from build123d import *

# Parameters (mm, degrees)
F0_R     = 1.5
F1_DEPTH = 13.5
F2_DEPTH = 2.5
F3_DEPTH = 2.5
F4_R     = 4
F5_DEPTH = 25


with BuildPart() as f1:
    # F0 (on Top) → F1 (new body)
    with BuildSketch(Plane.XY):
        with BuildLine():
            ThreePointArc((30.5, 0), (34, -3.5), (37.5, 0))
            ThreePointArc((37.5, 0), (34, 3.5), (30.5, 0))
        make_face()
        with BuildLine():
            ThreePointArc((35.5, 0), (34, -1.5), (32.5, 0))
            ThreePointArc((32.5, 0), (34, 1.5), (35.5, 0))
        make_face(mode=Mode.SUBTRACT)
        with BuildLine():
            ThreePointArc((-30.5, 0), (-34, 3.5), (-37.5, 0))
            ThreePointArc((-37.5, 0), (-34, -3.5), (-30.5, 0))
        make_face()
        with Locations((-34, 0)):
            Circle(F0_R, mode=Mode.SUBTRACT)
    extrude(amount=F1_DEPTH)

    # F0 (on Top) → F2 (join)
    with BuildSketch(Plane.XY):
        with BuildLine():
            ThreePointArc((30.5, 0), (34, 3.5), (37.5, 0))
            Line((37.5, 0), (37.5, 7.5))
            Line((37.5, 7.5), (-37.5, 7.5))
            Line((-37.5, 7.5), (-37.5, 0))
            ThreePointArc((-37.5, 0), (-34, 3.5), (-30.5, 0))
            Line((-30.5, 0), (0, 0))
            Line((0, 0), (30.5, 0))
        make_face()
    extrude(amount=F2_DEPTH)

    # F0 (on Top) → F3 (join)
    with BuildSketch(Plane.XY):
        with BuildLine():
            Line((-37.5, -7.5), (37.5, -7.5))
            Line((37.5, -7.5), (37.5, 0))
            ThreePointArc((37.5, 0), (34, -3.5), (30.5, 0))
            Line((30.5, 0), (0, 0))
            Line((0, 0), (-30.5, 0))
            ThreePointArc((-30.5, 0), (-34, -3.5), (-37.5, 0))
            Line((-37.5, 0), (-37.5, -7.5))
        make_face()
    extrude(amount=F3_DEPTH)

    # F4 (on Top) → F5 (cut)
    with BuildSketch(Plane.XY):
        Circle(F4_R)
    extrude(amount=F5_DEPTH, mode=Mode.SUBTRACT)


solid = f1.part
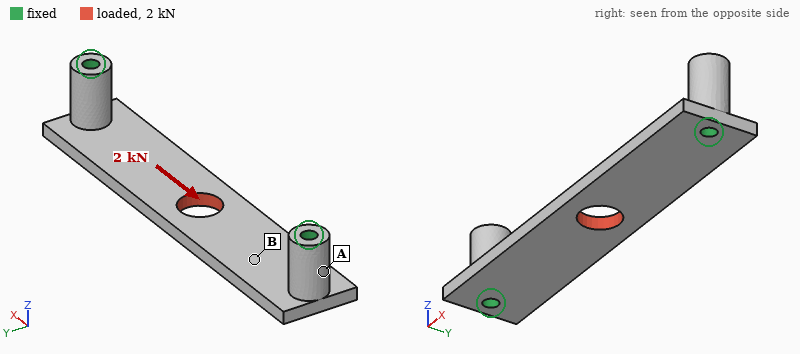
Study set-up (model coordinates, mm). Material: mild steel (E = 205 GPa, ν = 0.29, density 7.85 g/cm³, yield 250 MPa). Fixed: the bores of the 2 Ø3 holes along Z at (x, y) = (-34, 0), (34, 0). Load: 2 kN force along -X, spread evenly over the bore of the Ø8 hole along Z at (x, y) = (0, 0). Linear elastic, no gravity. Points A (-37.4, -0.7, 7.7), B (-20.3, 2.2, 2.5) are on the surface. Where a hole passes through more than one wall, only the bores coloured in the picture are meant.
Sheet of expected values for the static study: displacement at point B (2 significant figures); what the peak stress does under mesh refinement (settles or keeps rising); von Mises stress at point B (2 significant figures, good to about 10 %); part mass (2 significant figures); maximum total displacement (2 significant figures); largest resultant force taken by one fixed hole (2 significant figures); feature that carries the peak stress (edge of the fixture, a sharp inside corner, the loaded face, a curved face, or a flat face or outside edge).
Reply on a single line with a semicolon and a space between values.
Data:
2.3 µm; keeps rising; 29 MPa; 26 g; 5.0 µm; 1.0 kN; edge of the fixture
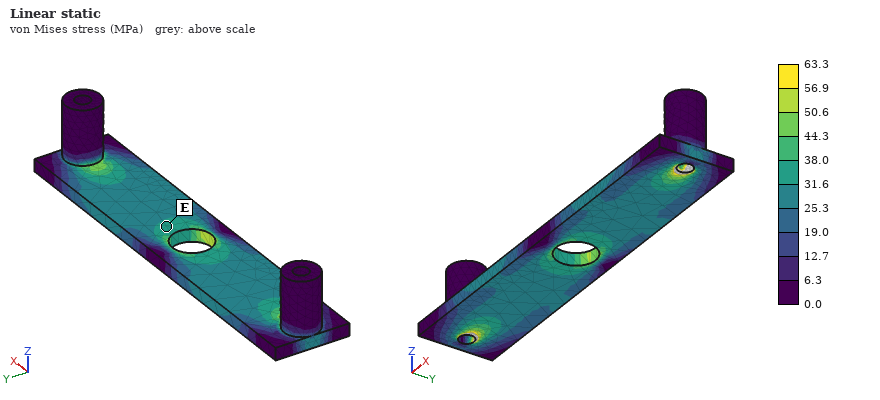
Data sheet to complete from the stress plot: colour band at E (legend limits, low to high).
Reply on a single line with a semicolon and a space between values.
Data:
31.6 to 38.0 MPa
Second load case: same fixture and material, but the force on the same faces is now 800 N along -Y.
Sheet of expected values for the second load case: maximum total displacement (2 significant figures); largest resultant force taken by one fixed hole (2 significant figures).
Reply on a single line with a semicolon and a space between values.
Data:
22 µm; 400 N
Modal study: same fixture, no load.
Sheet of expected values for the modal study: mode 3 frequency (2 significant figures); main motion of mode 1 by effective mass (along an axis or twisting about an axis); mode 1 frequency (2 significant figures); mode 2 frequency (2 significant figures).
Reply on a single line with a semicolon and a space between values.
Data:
8200 Hz; along Z; 3000 Hz; 7900 Hz
